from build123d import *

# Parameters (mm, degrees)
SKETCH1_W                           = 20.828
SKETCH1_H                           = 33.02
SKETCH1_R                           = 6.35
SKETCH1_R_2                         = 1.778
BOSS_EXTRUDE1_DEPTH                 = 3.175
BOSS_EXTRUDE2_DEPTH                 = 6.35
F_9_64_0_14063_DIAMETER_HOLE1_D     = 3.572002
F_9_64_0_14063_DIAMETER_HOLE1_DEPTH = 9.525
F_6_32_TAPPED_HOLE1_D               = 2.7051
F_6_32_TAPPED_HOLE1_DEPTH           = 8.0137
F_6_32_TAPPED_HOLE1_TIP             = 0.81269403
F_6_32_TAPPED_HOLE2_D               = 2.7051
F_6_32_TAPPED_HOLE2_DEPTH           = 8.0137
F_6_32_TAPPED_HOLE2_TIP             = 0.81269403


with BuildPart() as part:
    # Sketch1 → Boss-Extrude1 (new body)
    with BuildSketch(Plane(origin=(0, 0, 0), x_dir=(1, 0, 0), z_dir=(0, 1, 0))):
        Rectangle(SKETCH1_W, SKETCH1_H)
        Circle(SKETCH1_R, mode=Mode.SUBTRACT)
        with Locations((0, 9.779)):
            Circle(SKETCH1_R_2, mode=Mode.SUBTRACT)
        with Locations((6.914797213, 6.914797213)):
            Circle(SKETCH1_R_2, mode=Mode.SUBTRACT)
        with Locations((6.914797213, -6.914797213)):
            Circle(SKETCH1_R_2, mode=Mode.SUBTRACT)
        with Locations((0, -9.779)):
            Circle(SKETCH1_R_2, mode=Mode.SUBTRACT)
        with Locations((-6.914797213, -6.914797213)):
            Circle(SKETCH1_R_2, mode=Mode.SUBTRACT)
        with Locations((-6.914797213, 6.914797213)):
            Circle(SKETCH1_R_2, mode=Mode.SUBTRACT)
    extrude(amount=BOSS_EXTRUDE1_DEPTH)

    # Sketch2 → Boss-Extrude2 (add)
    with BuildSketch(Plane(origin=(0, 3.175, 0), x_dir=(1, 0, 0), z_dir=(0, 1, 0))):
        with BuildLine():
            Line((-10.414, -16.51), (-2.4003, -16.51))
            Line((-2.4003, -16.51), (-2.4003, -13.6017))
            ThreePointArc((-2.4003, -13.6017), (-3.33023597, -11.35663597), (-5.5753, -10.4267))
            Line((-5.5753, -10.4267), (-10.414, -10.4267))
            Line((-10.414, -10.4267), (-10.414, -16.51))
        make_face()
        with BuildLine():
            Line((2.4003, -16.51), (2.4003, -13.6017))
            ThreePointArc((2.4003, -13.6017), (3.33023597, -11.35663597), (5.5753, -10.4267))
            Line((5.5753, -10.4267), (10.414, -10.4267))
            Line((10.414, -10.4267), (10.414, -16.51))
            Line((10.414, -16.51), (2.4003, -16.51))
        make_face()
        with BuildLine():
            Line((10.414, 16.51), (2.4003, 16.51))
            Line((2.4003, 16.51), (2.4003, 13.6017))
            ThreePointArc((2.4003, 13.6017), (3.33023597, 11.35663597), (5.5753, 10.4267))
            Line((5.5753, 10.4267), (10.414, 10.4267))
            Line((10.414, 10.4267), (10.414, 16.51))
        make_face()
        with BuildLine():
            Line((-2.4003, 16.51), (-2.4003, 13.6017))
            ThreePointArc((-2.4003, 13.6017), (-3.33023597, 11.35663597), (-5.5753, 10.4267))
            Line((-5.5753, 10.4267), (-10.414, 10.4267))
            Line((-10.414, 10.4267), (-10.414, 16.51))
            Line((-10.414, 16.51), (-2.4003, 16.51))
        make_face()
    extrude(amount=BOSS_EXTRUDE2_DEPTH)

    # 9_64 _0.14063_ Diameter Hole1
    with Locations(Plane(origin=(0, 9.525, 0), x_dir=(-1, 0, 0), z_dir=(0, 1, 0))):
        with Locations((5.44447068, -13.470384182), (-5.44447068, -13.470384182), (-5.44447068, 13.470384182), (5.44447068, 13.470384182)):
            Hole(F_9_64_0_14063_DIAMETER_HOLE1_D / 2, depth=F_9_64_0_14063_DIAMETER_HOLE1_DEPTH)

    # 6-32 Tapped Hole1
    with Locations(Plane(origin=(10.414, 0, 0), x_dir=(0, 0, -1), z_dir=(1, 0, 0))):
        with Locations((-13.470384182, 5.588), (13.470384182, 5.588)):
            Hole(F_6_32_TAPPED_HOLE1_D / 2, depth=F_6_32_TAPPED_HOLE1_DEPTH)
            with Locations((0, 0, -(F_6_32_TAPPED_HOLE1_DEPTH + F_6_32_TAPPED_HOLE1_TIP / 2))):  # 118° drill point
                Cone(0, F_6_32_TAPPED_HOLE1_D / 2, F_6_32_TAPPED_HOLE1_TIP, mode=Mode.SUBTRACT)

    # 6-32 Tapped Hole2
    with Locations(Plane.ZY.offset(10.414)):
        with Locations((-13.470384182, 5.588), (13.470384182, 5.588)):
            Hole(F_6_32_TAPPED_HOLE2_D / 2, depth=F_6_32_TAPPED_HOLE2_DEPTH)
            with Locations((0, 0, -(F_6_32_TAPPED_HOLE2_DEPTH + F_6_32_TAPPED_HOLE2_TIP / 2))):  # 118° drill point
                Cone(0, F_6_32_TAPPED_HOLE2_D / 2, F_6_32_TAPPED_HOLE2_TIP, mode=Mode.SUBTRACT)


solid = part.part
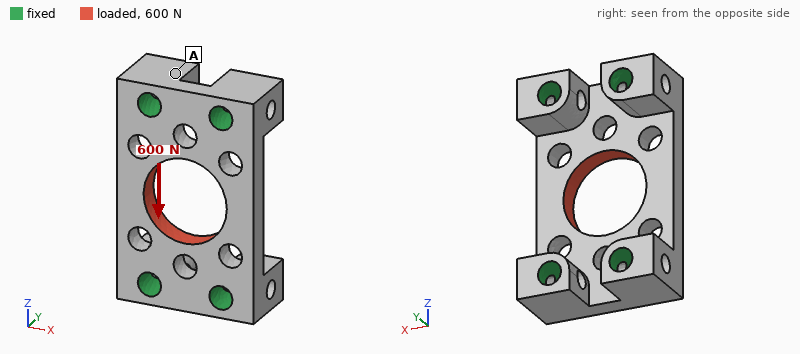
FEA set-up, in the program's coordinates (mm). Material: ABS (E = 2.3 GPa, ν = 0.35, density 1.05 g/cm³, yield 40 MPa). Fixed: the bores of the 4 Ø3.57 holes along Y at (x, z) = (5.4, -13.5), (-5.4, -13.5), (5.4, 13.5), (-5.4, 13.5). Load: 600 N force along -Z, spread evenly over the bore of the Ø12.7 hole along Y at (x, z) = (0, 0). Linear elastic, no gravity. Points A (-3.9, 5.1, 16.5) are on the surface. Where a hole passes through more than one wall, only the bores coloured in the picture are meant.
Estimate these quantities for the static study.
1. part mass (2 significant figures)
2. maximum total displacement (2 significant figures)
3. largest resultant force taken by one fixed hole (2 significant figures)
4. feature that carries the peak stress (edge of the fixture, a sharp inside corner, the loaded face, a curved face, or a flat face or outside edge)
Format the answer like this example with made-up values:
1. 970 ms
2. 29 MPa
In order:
1. 2.4 g
2. 49 µm
3. 150 N
4. a curved face
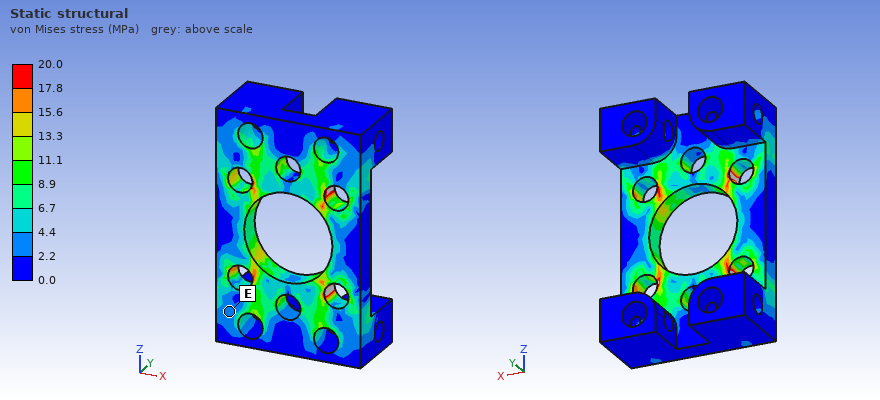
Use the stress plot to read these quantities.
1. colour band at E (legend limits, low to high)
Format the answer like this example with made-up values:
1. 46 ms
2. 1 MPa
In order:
1. 2.2 to 4.4 MPa
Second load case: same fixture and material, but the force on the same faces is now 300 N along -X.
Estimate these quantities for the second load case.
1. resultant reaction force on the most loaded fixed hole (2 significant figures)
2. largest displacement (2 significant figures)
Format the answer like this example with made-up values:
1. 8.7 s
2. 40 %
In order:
1. 80 N
2. 72 µm
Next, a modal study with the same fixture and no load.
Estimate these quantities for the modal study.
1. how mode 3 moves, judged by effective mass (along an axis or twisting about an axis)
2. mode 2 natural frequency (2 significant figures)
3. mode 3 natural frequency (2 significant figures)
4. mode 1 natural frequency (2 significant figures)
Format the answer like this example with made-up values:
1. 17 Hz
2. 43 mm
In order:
1. along X
2. 8700 Hz
3. 15 kHz
4. 8500 Hz
